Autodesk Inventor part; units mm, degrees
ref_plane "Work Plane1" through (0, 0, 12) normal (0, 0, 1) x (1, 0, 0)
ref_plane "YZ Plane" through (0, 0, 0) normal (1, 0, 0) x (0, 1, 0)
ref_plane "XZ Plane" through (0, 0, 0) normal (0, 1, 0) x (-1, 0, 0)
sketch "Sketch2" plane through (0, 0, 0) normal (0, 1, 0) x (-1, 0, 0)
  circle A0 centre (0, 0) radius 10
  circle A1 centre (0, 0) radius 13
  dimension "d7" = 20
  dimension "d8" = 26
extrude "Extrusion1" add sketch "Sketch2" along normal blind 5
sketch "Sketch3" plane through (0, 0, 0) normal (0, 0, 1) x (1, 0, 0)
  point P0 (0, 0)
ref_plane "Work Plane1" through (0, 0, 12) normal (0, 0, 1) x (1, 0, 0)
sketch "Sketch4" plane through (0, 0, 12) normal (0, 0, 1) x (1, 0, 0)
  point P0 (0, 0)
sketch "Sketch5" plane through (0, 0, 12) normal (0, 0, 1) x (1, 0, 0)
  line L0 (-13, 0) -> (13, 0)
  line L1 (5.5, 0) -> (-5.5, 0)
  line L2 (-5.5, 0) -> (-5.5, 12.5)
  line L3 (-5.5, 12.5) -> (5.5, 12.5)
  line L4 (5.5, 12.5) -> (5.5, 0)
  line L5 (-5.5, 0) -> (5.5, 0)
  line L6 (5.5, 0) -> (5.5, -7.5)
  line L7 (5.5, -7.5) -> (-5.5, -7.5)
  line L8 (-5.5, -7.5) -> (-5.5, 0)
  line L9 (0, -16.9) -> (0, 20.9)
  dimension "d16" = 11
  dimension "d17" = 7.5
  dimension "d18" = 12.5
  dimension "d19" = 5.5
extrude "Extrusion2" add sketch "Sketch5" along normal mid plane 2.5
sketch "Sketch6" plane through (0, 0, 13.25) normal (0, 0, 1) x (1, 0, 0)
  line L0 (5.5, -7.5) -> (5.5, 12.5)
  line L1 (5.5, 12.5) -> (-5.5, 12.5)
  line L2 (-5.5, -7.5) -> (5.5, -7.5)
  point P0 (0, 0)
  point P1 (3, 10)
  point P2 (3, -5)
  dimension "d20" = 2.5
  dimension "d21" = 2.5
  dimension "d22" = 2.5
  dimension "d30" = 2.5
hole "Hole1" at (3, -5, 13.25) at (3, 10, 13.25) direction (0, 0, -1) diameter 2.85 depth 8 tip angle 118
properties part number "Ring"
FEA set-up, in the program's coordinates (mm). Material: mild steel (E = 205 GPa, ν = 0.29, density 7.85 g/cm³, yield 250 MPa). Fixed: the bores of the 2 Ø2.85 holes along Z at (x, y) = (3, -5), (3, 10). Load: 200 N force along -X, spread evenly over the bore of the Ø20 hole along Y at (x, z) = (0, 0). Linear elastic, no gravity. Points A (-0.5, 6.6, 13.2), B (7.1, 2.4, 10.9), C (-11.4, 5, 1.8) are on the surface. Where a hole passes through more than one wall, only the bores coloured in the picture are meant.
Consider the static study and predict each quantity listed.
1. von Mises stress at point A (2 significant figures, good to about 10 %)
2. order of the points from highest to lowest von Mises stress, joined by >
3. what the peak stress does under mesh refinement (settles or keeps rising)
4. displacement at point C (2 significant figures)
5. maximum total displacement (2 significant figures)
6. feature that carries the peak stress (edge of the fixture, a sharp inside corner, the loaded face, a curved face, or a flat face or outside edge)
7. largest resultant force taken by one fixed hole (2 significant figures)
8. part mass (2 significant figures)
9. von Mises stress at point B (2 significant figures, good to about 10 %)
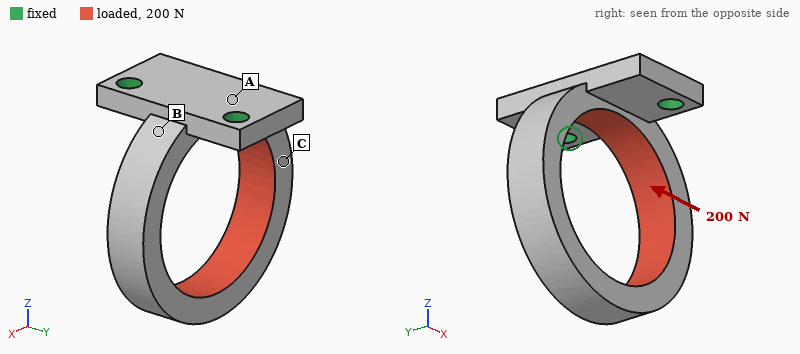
48 MPa
B > A > C
keeps rising
49 µm
83 µm
edge of the fixture
130 N
12 g
87 MPa
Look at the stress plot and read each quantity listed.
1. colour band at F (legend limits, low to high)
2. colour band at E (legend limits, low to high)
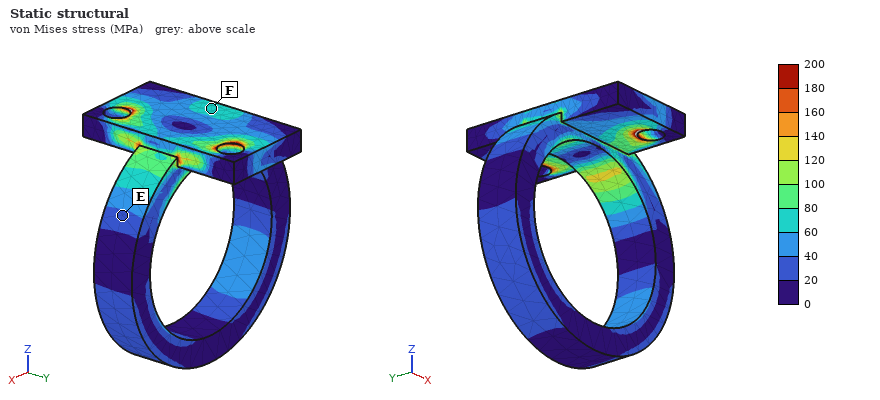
60 to 80 MPa
20 to 40 MPa
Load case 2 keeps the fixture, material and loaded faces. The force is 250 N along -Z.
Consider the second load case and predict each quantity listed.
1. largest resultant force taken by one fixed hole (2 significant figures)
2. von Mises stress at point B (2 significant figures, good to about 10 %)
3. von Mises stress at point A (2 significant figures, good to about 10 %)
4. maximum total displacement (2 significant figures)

130 N
16 MPa
28 MPa
16 µm
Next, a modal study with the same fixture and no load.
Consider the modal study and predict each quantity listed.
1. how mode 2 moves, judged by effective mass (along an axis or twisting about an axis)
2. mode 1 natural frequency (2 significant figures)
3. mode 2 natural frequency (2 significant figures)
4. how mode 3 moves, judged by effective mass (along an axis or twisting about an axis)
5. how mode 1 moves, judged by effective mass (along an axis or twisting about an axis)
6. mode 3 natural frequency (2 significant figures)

along Y
2900 Hz
3400 Hz
twisting about Z
along X
8800 Hz
